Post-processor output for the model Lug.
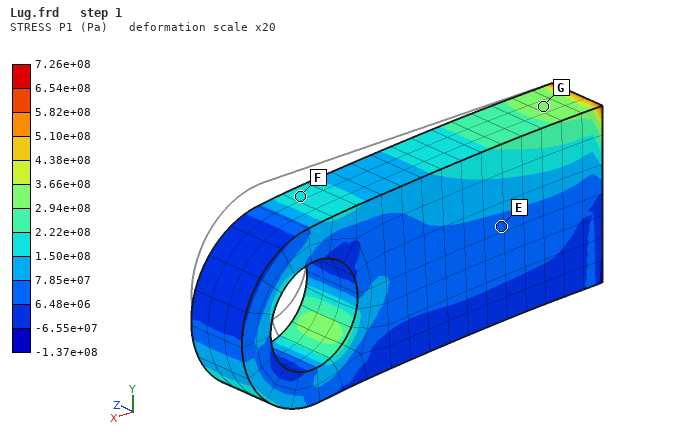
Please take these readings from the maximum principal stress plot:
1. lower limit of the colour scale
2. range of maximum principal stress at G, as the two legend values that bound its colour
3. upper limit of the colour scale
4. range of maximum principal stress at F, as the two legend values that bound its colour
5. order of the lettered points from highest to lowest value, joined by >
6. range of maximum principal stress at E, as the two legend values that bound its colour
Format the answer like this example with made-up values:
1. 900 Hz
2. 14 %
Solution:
1. -1.37e+08 Pa
2. 2.94e+08 to 3.66e+08 Pa
3. 7.26e+08 Pa
4. 1.50e+08 to 2.22e+08 Pa
5. G > F > E
6. 6.48e+06 to 7.85e+07 Pa
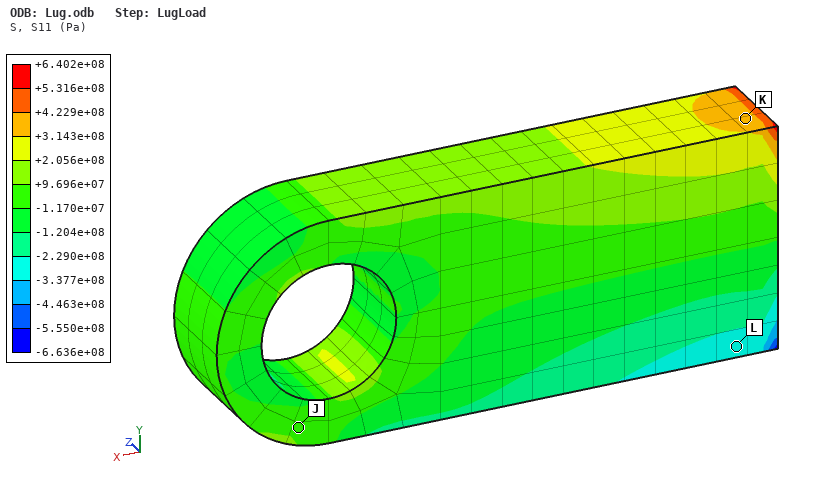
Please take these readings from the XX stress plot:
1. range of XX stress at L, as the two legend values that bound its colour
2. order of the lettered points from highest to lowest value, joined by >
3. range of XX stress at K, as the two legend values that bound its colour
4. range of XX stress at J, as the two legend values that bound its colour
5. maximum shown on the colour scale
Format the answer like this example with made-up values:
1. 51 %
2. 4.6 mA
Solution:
1. -3.377e+08 to -2.290e+08 Pa
2. K > J > L
3. +3.143e+08 to +4.229e+08 Pa
4. -1.170e+07 to +9.696e+07 Pa
5. +6.402e+08 Pa
